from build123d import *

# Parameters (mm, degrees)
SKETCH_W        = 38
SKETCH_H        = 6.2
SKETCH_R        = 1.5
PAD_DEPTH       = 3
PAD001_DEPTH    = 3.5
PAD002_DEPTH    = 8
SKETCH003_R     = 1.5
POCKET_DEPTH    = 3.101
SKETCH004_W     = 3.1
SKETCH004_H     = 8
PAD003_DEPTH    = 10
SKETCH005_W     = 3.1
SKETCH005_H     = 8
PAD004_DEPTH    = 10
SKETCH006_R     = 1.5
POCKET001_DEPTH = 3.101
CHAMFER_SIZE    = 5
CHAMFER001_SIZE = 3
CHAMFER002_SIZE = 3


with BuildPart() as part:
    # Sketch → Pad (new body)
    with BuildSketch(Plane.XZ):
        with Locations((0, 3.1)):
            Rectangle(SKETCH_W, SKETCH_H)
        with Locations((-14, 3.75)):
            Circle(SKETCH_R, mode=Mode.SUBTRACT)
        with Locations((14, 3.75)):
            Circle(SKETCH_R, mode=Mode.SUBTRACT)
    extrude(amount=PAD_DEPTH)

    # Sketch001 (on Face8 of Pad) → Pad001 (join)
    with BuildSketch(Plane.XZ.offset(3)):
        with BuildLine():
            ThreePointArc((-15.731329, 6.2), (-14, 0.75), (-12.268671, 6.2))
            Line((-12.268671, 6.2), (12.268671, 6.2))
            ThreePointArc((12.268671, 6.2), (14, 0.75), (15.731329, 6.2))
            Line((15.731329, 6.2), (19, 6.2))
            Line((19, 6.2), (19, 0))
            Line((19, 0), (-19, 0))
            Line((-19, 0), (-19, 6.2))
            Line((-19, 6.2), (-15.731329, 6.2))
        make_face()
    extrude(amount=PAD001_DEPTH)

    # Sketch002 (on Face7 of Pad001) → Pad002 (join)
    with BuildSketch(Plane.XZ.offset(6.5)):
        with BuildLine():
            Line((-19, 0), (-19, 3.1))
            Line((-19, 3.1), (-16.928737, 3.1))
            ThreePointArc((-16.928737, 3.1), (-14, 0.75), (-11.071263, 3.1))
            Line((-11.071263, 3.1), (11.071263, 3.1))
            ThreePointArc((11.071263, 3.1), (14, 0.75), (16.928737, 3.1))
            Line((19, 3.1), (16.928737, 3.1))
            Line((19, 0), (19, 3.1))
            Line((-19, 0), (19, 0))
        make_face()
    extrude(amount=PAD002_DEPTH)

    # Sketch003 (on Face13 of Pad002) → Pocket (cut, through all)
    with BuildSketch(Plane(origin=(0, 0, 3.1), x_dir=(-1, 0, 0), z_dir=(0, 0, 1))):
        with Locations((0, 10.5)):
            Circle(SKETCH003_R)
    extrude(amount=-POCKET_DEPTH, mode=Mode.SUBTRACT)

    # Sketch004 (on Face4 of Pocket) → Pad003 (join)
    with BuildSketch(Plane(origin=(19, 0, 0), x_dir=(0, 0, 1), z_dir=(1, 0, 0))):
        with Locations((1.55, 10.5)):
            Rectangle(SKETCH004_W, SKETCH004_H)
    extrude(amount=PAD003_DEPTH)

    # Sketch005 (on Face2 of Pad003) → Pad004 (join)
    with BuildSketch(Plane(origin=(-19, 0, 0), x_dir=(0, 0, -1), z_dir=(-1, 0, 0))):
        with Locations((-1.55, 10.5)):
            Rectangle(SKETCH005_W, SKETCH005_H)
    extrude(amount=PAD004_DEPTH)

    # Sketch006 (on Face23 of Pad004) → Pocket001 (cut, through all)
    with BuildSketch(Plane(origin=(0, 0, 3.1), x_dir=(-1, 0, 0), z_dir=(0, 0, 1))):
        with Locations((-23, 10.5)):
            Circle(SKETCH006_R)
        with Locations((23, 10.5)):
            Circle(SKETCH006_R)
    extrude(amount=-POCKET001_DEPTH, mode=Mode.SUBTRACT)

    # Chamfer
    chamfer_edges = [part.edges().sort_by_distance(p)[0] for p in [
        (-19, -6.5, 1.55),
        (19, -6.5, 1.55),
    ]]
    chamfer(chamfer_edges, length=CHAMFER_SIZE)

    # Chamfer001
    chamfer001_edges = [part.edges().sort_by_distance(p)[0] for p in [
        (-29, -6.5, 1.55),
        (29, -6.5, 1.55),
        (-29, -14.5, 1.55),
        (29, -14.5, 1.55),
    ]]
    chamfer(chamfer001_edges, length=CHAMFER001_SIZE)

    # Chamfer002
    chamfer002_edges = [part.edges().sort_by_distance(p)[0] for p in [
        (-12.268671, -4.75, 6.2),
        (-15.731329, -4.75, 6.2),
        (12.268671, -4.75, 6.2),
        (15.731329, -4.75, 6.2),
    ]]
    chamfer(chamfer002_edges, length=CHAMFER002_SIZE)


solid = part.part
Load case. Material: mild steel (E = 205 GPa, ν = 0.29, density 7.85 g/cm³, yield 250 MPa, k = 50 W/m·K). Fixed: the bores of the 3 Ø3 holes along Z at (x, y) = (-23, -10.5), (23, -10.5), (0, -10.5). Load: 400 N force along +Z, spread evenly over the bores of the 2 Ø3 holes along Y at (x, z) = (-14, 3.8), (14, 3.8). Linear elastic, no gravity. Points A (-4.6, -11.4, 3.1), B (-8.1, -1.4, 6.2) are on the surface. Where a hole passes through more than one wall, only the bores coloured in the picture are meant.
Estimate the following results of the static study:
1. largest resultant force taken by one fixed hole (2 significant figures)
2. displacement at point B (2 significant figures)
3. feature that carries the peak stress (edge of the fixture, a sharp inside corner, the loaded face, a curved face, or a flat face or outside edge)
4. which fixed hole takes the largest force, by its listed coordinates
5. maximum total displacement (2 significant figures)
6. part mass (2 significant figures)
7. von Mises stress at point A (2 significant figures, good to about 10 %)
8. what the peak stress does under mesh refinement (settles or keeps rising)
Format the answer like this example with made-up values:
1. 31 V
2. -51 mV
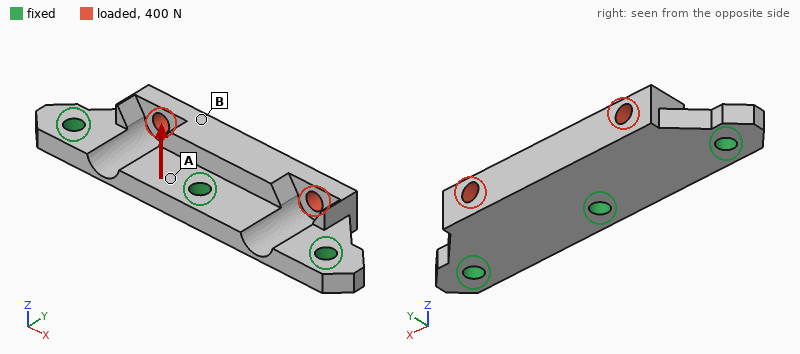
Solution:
1. 210 N
2. 8.2 µm
3. edge of the fixture
4. (0, -10.5)
5. 10 µm
6. 20 g
7. 25 MPa
8. keeps rising
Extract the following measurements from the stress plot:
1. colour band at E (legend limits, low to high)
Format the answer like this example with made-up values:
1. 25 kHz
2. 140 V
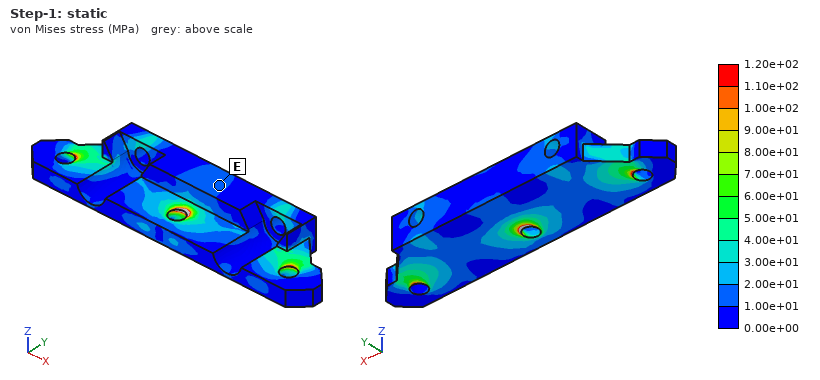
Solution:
1. 1.00e+01 to 2.00e+01 MPa
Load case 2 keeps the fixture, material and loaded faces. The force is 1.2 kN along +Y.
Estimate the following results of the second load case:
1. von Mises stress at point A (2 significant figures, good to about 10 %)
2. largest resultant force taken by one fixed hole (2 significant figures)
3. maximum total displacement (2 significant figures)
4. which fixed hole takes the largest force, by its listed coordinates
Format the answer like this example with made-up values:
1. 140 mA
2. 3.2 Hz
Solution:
1. 34 MPa
2. 590 N
3. 13 µm
4. (0, -10.5)
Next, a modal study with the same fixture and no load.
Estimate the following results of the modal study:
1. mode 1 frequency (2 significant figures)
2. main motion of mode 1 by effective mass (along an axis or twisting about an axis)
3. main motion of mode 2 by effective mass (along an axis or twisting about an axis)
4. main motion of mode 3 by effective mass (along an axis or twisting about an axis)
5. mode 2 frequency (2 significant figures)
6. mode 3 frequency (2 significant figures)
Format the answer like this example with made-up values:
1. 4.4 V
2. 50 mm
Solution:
1. 13 kHz
2. along Z
3. twisting about Y
4. along Z
5. 19 kHz
6. 35 kHz
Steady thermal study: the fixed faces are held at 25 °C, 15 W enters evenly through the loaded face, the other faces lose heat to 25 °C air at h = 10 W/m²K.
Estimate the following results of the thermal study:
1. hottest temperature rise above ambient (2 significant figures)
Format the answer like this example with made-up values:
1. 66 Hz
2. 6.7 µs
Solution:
1. 48 K
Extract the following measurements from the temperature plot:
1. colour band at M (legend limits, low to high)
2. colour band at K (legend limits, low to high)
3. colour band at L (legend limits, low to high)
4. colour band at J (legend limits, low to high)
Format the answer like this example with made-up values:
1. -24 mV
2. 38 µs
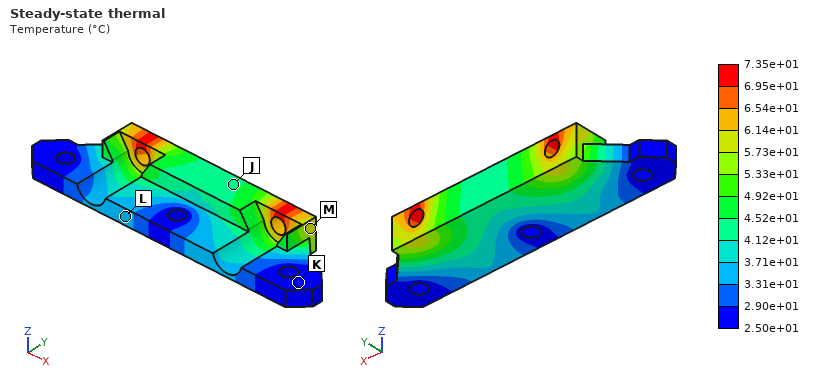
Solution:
1. 5.73e+01 to 6.14e+01 °C
2. 2.50e+01 to 2.90e+01 °C
3. 3.31e+01 to 3.71e+01 °C
4. 4.12e+01 to 4.52e+01 °C
